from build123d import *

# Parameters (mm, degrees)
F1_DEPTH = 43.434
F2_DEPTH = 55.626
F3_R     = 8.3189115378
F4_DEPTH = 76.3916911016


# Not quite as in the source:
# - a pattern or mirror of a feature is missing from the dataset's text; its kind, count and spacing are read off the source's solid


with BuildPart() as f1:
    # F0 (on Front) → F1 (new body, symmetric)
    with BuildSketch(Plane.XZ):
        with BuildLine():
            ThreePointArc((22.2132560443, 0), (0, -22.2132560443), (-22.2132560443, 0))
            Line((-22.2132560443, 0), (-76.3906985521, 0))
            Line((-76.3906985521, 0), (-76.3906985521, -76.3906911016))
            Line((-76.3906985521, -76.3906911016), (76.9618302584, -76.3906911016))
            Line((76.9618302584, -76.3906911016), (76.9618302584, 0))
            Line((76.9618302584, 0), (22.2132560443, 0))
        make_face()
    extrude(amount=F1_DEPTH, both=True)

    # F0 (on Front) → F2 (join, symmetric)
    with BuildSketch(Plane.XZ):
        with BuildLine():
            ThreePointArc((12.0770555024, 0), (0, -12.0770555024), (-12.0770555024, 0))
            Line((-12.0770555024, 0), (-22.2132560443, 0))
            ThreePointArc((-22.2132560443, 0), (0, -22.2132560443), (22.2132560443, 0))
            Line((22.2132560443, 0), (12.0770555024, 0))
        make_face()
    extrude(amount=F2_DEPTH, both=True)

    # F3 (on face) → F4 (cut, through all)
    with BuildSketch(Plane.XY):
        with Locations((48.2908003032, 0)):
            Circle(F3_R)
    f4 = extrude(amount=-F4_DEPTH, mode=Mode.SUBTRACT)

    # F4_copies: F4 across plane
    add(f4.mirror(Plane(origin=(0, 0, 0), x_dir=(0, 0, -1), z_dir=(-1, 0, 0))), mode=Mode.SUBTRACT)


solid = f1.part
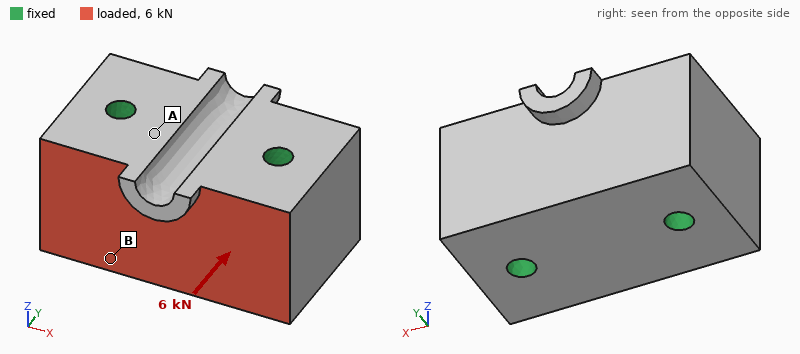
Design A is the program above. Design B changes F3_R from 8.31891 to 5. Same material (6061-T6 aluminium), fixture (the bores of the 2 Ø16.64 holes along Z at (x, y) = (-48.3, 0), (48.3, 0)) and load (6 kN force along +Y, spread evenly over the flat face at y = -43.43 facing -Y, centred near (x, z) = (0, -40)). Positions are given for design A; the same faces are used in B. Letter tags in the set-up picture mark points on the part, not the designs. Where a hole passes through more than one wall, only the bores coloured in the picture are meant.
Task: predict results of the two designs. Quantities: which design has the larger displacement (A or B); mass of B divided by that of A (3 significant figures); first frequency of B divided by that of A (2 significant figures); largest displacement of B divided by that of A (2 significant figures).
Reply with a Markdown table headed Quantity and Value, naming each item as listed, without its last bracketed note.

| Quantity | Value |
|---|---|
| which design has the larger displacement | B |
| mass of B divided by that of A | 1.02 |
| first frequency of B divided by that of A | 0.85 |
| largest displacement of B divided by that of A | 1.2 |
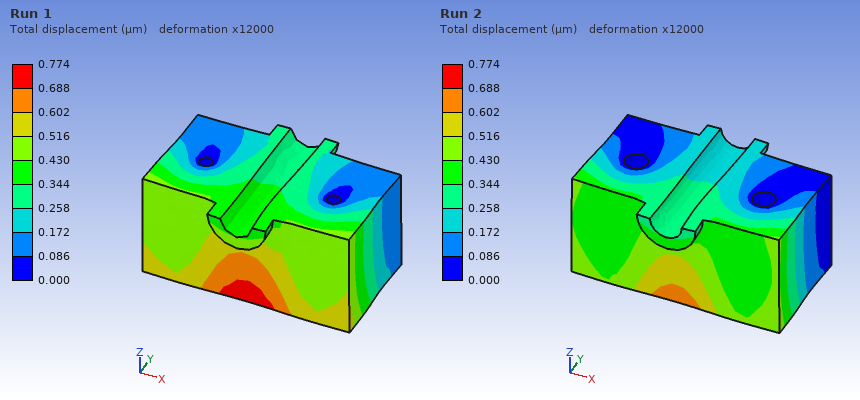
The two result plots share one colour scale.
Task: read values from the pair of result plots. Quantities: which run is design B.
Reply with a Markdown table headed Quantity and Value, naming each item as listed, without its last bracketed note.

| Quantity | Value |
|---|---|
| which run is design B | Run 1 |
